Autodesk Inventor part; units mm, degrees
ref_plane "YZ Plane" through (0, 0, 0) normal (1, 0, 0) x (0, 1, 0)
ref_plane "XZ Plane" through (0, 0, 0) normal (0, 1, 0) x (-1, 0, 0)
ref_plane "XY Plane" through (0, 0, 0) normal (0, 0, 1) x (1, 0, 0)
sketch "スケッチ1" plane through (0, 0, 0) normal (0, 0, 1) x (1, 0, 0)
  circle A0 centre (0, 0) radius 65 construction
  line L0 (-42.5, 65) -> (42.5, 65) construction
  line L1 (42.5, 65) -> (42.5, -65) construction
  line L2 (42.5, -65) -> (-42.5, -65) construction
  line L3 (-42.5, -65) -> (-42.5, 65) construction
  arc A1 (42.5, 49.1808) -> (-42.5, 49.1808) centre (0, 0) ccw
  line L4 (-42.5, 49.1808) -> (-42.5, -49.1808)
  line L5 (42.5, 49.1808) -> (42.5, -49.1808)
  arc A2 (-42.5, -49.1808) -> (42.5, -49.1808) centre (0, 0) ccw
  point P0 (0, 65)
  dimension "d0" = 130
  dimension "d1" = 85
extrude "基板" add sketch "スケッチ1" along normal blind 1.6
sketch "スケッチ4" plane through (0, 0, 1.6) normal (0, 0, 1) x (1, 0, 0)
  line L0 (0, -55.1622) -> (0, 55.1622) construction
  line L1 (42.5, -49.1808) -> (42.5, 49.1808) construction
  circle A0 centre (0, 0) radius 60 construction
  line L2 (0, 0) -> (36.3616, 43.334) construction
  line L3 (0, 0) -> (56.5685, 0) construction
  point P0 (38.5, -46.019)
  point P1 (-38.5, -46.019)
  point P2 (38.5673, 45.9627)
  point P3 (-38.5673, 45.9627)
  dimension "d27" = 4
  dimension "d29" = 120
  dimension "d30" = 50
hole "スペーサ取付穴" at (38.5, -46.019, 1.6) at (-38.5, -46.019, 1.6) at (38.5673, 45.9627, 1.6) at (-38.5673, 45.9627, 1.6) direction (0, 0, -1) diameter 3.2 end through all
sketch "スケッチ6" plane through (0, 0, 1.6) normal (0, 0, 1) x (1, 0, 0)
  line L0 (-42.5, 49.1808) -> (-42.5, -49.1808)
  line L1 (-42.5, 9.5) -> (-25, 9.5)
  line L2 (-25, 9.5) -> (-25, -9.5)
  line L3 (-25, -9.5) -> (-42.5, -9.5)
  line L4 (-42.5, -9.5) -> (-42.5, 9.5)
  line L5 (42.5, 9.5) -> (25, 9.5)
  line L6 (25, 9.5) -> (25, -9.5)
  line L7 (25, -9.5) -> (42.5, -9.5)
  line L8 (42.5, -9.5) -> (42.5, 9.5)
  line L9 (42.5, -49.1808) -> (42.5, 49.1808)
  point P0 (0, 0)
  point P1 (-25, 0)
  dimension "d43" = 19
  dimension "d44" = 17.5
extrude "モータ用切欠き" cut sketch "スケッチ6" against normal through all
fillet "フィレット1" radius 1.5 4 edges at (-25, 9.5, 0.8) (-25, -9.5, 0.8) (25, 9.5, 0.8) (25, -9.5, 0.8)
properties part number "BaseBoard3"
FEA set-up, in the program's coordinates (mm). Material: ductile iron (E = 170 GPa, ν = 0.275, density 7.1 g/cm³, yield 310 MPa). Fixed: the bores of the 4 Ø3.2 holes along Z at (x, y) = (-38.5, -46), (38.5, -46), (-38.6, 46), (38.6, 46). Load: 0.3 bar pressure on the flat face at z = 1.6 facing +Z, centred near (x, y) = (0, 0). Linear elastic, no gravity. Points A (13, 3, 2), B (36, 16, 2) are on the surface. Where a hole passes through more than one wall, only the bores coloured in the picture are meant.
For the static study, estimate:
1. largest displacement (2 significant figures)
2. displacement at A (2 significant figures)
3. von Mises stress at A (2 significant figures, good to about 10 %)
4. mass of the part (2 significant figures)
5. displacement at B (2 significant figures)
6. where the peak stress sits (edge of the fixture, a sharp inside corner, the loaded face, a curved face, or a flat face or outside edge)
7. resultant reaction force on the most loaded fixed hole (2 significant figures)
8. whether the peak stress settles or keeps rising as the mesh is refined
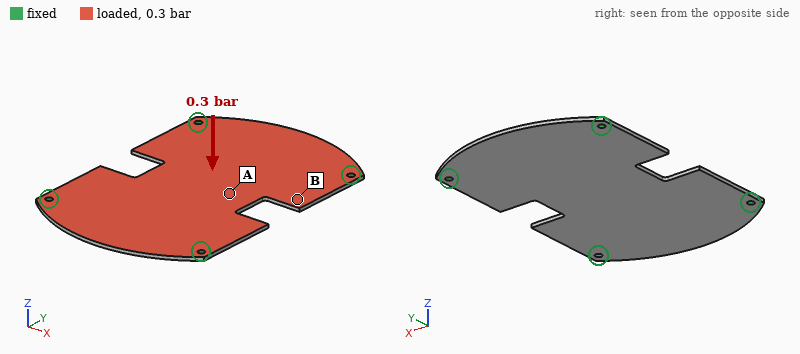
0.22 mm
0.21 mm
31 MPa
110 g
0.13 mm
edge of the fixture
71 N
keeps rising
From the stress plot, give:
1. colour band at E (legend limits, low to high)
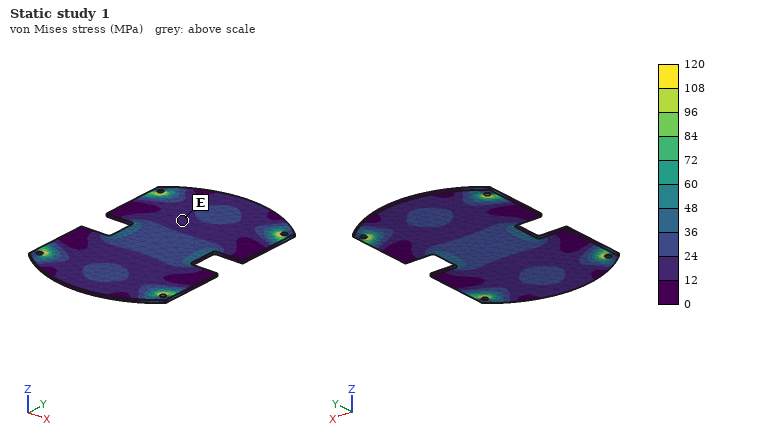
12 to 24 MPa
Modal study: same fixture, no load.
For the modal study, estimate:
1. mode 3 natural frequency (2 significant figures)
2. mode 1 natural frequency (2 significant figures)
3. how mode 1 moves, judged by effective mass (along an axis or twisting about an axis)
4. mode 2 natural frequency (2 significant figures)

1200 Hz
660 Hz
along Z
1200 Hz
